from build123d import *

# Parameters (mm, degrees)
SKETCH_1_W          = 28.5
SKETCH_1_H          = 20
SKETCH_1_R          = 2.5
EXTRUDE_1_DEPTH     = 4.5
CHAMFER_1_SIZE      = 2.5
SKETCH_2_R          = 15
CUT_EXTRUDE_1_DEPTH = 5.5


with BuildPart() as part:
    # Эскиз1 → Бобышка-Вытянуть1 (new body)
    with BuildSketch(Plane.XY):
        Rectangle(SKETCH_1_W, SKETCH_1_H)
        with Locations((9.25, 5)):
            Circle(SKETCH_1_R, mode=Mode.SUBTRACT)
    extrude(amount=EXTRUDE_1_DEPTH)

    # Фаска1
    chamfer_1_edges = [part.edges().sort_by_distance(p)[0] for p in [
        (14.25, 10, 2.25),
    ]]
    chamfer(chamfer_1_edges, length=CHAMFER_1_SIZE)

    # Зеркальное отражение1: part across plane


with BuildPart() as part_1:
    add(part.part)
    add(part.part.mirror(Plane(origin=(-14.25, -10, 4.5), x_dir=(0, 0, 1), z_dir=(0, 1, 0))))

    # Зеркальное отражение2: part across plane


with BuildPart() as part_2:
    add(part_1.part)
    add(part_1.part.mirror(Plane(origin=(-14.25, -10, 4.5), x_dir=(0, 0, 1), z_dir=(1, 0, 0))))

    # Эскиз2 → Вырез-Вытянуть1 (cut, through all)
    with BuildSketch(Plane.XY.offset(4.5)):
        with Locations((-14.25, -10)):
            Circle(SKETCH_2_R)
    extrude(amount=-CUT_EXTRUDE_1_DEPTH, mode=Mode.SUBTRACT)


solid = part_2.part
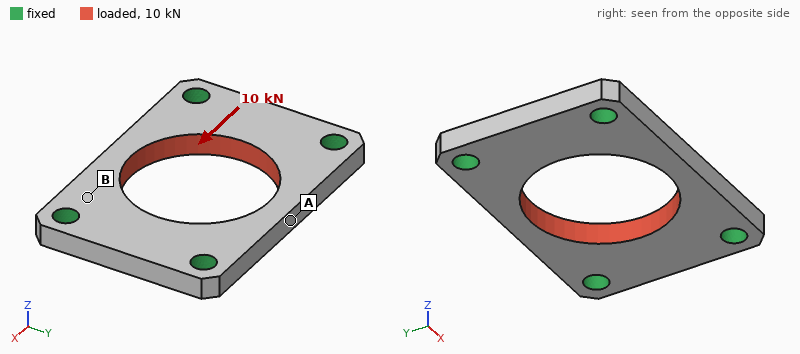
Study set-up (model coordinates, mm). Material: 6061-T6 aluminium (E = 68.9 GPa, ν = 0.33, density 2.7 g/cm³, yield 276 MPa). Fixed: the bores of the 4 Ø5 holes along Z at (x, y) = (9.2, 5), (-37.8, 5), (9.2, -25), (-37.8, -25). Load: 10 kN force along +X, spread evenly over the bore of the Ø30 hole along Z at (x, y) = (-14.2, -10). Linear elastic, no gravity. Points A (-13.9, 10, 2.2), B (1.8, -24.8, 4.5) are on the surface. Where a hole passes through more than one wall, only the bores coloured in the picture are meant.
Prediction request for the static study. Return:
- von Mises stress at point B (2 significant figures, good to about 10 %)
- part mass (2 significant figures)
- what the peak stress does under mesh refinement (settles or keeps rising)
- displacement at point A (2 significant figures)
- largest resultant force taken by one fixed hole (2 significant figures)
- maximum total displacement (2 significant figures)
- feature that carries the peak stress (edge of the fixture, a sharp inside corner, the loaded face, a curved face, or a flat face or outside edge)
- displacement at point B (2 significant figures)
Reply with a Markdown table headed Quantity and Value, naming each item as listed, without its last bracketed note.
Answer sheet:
| Quantity | Value |
|---|---|
| von Mises stress at point B | 42 MPa |
| part mass | 18 g |
| what the peak stress does under mesh refinement | keeps rising |
| displacement at point A | 8.5 µm |
| largest resultant force taken by one fixed hole | 2.6 kN |
| maximum total displacement | 12 µm |
| feature that carries the peak stress | edge of the fixture |
| displacement at point B | 3.7 µm |
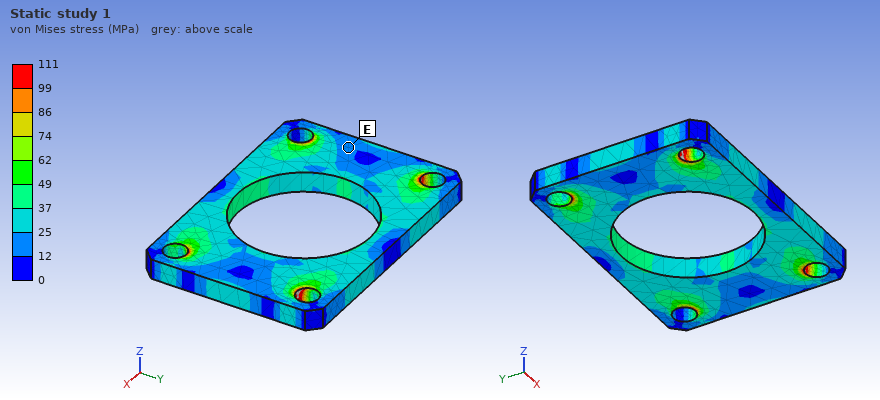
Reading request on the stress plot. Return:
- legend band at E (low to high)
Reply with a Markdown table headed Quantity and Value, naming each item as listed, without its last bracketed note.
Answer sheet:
| Quantity | Value |
|---|---|
| legend band at E | 12 to 25 MPa |
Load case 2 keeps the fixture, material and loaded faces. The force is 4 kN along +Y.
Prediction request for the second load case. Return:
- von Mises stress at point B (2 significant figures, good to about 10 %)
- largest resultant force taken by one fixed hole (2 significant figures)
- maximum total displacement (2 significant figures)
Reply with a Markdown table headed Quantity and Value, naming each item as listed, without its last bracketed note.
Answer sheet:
| Quantity | Value |
|---|---|
| von Mises stress at point B | 13 MPa |
| largest resultant force taken by one fixed hole | 1.0 kN |
| maximum total displacement | 21 µm |
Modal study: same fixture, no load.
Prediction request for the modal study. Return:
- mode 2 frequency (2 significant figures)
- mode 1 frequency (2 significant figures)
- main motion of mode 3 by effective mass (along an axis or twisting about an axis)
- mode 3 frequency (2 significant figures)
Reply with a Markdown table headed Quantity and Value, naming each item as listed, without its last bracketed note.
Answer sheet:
| Quantity | Value |
|---|---|
| mode 2 frequency | 14 kHz |
| mode 1 frequency | 13 kHz |
| main motion of mode 3 by effective mass | twisting about Y |
| mode 3 frequency | 23 kHz |
